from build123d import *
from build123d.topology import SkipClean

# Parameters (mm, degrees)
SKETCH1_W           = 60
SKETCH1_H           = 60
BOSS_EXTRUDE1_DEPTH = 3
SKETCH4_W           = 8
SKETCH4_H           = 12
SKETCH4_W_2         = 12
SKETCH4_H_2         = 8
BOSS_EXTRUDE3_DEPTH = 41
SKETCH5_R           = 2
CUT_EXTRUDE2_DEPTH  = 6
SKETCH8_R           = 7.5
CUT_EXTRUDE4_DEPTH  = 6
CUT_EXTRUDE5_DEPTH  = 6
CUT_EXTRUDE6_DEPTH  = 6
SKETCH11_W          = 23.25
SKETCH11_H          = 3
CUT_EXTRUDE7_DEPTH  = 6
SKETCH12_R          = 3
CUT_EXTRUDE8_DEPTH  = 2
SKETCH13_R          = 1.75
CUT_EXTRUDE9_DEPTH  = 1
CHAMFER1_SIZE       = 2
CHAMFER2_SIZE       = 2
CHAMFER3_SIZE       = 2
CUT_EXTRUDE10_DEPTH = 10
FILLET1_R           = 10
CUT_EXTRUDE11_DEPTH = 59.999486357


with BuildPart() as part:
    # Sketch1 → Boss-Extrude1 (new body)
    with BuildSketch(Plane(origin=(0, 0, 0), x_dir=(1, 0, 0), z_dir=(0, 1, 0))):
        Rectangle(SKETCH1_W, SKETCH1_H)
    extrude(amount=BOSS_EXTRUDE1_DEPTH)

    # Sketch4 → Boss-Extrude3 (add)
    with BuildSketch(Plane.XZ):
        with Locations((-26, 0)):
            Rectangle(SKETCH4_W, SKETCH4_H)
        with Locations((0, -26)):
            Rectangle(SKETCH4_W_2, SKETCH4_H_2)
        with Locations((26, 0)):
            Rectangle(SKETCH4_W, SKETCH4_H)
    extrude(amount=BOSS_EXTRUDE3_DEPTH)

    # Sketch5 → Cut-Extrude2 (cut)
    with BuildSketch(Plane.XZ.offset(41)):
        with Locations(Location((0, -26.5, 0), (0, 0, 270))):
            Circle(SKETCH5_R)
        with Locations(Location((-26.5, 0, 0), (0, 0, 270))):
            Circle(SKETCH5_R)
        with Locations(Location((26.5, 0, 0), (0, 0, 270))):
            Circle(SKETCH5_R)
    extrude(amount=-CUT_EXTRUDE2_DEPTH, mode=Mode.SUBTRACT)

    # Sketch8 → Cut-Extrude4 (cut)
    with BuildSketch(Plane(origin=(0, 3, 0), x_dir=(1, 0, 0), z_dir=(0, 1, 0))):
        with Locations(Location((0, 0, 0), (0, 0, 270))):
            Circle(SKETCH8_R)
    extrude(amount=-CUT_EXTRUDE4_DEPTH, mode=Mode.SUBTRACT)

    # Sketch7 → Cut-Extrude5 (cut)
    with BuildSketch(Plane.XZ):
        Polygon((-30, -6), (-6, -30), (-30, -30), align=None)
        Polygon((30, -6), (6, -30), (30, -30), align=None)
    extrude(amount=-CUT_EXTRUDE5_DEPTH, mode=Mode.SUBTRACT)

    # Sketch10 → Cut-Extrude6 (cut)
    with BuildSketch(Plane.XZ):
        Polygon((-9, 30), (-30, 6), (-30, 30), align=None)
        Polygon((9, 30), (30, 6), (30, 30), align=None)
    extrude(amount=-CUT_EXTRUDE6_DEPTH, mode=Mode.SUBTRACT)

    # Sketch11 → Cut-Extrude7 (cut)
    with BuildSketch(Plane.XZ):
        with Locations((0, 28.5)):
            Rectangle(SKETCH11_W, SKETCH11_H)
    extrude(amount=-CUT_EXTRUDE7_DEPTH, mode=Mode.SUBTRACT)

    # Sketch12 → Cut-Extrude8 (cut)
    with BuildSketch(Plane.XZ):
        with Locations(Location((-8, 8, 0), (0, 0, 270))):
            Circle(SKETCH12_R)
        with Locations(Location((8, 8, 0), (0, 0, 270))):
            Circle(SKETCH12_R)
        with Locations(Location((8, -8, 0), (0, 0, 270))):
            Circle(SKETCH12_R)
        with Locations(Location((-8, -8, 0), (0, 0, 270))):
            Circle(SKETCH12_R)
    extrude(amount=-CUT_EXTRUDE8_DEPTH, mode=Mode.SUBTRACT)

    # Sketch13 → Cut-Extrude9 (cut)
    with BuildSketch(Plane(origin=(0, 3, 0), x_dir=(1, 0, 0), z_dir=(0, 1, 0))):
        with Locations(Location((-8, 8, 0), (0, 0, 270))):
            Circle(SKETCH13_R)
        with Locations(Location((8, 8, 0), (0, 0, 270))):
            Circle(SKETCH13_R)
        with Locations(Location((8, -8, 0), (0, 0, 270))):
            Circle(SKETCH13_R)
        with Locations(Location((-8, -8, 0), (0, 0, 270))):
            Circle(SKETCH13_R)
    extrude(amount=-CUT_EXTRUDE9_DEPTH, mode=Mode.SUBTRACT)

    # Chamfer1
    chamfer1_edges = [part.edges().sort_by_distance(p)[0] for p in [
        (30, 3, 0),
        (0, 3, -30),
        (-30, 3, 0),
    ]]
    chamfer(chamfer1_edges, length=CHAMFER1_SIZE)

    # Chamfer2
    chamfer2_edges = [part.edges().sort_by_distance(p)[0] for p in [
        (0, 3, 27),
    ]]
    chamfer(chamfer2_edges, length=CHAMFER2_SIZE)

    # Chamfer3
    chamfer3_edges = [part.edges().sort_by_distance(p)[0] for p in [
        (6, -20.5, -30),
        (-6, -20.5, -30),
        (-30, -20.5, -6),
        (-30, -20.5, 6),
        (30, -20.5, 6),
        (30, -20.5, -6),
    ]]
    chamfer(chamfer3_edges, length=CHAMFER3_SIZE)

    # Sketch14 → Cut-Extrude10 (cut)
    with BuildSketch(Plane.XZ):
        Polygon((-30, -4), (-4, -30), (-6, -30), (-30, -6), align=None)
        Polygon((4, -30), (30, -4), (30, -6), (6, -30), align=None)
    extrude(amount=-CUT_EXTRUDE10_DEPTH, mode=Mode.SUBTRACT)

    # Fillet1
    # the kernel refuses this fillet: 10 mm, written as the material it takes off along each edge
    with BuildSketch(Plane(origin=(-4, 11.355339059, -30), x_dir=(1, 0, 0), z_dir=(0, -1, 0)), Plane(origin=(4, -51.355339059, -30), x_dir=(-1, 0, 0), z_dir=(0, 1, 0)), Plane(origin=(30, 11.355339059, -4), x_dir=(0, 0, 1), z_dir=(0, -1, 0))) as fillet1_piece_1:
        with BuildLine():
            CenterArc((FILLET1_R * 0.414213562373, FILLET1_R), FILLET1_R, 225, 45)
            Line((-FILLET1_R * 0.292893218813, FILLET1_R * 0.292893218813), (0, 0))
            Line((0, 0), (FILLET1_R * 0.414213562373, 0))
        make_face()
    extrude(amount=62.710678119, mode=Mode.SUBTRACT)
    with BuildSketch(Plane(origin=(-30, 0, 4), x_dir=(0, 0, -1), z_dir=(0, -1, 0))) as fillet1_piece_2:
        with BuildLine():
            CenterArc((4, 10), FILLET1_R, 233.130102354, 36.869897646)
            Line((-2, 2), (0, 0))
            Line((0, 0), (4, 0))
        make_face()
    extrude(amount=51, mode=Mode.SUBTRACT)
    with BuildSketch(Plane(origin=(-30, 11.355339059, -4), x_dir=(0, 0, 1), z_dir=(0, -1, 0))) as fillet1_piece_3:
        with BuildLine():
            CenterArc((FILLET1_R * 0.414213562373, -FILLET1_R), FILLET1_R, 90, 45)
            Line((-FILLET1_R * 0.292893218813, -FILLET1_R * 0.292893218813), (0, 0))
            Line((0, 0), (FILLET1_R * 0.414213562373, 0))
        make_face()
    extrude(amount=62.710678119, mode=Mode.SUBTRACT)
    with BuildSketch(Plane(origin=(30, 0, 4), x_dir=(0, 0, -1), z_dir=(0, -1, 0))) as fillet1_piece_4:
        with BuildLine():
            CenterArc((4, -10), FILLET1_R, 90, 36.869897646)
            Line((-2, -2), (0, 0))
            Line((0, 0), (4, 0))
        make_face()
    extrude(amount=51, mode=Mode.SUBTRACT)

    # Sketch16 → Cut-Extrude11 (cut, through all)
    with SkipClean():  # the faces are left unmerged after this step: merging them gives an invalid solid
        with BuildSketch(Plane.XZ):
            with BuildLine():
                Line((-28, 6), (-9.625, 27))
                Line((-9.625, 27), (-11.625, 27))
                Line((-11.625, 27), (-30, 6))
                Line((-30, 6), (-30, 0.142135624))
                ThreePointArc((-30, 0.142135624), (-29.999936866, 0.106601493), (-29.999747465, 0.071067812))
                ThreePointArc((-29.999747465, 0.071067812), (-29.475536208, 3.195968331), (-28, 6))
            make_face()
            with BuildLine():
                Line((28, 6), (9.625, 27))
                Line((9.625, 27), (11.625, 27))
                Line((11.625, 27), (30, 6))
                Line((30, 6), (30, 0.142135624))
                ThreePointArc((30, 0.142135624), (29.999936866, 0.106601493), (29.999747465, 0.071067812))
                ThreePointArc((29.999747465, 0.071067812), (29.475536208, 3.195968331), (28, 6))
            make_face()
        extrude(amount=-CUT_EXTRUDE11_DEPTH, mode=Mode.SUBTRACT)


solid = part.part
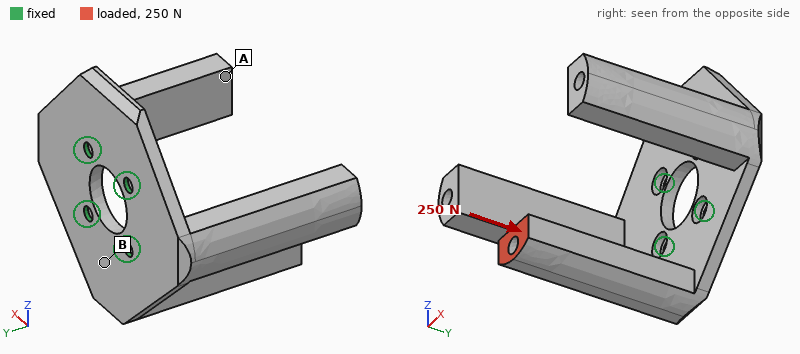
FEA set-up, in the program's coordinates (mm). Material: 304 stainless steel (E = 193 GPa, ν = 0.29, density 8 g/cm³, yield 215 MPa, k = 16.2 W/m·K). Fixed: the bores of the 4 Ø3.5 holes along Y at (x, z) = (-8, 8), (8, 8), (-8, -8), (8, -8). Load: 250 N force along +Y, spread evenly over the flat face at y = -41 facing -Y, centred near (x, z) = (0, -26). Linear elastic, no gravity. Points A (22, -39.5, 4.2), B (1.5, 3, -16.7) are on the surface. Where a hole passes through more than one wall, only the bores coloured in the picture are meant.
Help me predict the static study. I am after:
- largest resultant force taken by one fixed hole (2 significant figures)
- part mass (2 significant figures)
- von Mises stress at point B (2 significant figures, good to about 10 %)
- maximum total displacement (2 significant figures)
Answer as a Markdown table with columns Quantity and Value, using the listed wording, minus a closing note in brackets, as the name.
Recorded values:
| Quantity | Value |
|---|---|
| largest resultant force taken by one fixed hole | 310 N |
| part mass | 130 g |
| von Mises stress at point B | 42 MPa |
| maximum total displacement | 0.18 mm |
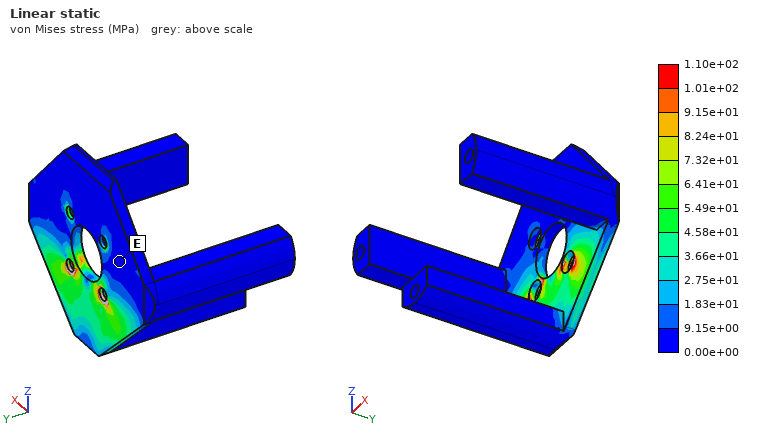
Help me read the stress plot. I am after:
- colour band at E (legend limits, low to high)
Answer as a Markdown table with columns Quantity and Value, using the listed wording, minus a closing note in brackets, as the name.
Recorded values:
| Quantity | Value |
|---|---|
| colour band at E | 0.00e+00 to 9.15e+00 MPa |
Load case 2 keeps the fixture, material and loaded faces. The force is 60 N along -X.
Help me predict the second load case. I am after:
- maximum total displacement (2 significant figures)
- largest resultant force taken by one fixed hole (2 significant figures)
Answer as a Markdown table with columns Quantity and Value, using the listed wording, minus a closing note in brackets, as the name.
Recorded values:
| Quantity | Value |
|---|---|
| maximum total displacement | 68 µm |
| largest resultant force taken by one fixed hole | 220 N |
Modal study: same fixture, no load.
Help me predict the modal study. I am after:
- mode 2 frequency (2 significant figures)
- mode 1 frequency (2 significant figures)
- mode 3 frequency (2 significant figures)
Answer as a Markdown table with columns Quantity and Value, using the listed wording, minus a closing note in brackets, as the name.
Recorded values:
| Quantity | Value |
|---|---|
| mode 2 frequency | 870 Hz |
| mode 1 frequency | 830 Hz |
| mode 3 frequency | 900 Hz |
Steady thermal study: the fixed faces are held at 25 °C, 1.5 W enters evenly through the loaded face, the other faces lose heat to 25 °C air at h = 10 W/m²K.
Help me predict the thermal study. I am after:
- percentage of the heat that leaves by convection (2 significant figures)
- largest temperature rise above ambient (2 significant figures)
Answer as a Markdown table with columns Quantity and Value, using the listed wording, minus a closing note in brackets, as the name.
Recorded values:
| Quantity | Value |
|---|---|
| percentage of the heat that leaves by convection | 45 % |
| largest temperature rise above ambient | 50 K |
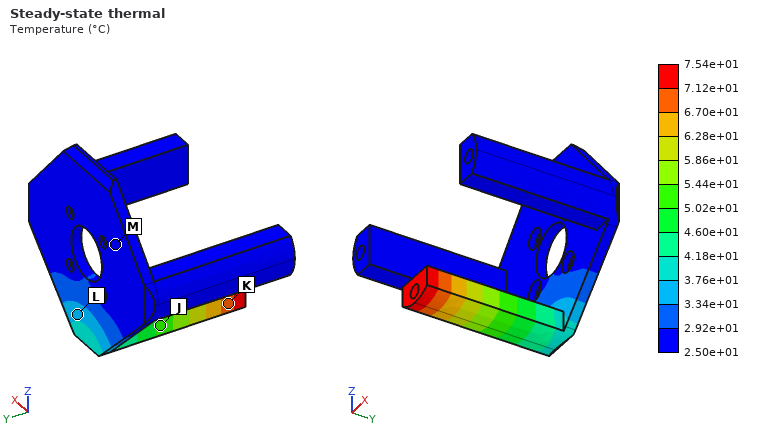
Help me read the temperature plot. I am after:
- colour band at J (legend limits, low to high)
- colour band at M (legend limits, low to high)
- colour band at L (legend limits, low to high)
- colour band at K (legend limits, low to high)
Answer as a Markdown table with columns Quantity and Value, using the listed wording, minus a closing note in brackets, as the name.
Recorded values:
| Quantity | Value |
|---|---|
| colour band at J | 5.02e+01 to 5.44e+01 °C |
| colour band at M | 2.50e+01 to 2.92e+01 °C |
| colour band at L | 3.34e+01 to 3.76e+01 °C |
| colour band at K | 6.70e+01 to 7.12e+01 °C |
